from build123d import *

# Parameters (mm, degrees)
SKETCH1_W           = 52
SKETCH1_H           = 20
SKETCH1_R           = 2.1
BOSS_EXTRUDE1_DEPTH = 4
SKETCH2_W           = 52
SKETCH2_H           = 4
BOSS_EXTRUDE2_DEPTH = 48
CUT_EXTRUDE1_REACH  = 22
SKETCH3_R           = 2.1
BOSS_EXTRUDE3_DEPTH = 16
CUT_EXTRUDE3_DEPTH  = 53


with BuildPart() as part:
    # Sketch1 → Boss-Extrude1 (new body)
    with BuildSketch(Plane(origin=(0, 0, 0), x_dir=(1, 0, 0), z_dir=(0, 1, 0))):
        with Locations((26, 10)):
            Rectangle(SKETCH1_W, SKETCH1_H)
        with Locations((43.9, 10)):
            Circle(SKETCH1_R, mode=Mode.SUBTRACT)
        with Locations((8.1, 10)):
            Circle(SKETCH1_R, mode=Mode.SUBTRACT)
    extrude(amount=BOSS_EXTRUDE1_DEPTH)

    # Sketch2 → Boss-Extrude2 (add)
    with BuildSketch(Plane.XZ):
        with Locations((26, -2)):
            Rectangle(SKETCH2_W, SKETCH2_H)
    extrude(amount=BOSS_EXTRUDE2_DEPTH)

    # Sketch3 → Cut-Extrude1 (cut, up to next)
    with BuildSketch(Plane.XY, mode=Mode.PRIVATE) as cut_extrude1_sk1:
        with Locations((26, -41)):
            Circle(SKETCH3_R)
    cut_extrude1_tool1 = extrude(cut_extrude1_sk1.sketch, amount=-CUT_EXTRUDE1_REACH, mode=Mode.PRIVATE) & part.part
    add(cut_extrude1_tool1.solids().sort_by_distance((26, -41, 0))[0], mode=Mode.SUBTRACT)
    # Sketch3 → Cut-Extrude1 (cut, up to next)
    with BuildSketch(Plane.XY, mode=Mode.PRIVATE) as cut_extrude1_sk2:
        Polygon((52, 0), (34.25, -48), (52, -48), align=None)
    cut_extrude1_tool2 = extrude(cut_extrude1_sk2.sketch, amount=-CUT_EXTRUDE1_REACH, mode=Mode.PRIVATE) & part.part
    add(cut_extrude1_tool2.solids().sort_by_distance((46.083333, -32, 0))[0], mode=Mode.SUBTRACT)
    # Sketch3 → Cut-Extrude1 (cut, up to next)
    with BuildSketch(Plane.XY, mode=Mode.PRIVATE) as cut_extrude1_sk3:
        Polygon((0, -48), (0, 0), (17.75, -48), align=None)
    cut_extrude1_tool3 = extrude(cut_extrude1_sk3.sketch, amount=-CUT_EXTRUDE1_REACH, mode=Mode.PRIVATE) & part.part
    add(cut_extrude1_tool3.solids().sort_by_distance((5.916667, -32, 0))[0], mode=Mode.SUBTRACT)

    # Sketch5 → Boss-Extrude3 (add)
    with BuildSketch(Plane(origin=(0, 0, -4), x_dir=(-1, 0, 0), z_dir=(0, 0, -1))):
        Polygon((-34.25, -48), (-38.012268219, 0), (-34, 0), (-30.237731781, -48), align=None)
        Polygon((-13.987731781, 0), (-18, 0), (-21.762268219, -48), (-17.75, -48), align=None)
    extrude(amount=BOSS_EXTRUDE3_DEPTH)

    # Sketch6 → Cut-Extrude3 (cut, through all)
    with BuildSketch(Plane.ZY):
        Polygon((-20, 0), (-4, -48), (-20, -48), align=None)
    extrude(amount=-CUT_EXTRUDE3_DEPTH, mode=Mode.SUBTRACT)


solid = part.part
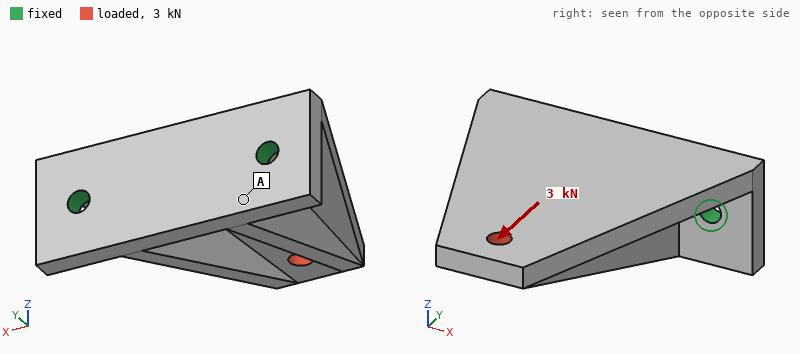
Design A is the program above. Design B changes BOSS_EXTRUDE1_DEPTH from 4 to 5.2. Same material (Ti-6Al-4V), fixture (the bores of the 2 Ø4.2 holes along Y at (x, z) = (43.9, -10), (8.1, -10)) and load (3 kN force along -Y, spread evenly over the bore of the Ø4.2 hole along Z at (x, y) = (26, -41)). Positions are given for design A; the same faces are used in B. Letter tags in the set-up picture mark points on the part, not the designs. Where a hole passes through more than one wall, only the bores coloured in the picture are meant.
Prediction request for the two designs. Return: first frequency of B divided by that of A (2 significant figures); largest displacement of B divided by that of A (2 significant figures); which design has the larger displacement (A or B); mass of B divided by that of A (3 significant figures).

1.2
0.66
A
1.09
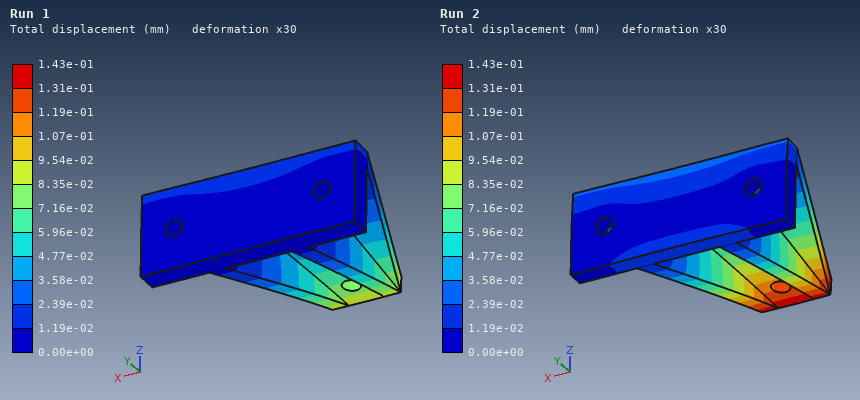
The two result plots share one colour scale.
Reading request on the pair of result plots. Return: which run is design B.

Run 1
